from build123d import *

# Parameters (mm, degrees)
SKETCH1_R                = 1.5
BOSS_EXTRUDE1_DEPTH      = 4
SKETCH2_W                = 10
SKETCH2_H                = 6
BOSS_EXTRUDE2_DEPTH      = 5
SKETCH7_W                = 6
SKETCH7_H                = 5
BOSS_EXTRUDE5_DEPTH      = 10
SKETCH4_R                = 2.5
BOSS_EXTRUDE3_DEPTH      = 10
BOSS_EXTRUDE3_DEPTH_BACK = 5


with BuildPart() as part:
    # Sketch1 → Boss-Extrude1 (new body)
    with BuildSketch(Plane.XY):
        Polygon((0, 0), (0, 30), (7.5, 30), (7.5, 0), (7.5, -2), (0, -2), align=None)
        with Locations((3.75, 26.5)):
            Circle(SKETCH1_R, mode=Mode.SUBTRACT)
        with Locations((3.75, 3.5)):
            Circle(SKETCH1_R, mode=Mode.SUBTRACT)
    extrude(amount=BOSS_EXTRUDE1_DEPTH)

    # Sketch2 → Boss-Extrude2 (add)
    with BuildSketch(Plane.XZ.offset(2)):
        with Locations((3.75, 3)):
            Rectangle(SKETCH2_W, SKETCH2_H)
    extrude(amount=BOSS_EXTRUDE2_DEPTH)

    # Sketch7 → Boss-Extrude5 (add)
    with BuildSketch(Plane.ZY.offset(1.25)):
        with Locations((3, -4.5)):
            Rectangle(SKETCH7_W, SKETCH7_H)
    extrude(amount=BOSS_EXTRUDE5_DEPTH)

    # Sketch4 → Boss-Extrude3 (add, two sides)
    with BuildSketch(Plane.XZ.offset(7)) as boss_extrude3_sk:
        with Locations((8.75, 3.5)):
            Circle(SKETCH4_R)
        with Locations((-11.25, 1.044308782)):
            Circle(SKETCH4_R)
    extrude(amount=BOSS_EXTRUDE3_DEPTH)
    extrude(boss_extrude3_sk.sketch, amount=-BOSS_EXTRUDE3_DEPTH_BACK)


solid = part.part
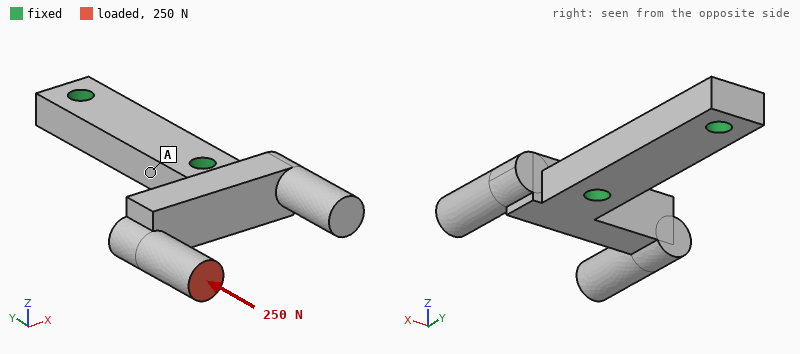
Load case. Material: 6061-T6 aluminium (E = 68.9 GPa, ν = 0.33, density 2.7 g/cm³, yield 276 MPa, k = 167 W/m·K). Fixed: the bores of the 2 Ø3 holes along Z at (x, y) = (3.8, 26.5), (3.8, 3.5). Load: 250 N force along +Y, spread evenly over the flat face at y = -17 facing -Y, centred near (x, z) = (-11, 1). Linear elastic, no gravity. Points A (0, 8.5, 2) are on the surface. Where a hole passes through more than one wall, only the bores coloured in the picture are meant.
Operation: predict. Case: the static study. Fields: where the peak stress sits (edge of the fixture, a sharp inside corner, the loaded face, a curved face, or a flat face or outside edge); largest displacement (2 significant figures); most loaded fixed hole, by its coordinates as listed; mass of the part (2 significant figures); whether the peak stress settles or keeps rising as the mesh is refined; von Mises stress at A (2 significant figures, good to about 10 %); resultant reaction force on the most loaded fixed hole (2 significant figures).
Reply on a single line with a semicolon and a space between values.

a sharp inside corner; 0.19 mm; (3.8, 3.5); 5.4 g; keeps rising; 17 MPa; 250 N
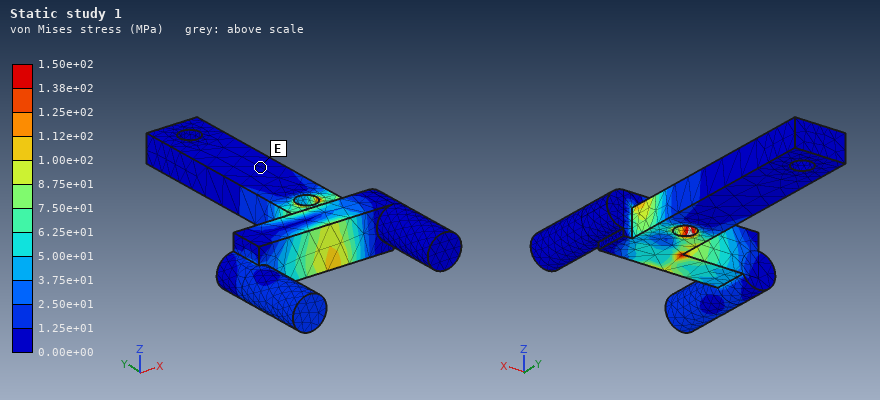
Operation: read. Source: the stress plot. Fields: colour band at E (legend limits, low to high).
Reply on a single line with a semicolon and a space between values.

0.00e+00 to 1.25e+01 MPa
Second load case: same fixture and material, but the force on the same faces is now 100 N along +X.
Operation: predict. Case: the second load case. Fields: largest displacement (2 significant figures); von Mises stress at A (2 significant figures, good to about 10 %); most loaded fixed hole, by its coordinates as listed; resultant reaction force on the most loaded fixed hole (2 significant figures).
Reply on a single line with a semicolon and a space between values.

0.13 mm; 8.6 MPa; (3.8, 3.5); 130 N
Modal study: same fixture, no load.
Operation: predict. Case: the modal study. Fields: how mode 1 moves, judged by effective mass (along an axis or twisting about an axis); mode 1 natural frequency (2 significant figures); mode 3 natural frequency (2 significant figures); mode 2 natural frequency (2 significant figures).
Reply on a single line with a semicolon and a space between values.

along Z; 5000 Hz; 8500 Hz; 6000 Hz
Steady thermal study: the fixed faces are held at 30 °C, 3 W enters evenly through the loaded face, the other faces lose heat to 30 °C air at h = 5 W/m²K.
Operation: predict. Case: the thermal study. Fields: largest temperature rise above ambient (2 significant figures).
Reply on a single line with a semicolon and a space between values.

22 K
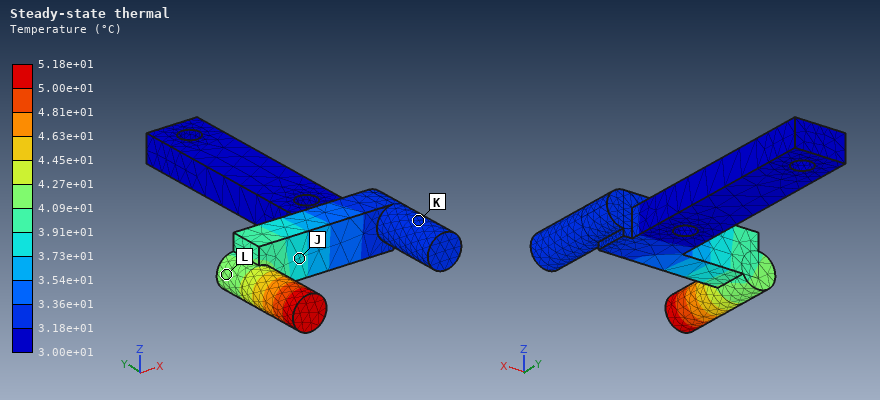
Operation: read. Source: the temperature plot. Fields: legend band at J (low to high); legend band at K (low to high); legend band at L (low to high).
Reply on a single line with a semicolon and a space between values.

3.73e+01 to 3.91e+01 °C; 3.18e+01 to 3.36e+01 °C; 4.09e+01 to 4.27e+01 °C
